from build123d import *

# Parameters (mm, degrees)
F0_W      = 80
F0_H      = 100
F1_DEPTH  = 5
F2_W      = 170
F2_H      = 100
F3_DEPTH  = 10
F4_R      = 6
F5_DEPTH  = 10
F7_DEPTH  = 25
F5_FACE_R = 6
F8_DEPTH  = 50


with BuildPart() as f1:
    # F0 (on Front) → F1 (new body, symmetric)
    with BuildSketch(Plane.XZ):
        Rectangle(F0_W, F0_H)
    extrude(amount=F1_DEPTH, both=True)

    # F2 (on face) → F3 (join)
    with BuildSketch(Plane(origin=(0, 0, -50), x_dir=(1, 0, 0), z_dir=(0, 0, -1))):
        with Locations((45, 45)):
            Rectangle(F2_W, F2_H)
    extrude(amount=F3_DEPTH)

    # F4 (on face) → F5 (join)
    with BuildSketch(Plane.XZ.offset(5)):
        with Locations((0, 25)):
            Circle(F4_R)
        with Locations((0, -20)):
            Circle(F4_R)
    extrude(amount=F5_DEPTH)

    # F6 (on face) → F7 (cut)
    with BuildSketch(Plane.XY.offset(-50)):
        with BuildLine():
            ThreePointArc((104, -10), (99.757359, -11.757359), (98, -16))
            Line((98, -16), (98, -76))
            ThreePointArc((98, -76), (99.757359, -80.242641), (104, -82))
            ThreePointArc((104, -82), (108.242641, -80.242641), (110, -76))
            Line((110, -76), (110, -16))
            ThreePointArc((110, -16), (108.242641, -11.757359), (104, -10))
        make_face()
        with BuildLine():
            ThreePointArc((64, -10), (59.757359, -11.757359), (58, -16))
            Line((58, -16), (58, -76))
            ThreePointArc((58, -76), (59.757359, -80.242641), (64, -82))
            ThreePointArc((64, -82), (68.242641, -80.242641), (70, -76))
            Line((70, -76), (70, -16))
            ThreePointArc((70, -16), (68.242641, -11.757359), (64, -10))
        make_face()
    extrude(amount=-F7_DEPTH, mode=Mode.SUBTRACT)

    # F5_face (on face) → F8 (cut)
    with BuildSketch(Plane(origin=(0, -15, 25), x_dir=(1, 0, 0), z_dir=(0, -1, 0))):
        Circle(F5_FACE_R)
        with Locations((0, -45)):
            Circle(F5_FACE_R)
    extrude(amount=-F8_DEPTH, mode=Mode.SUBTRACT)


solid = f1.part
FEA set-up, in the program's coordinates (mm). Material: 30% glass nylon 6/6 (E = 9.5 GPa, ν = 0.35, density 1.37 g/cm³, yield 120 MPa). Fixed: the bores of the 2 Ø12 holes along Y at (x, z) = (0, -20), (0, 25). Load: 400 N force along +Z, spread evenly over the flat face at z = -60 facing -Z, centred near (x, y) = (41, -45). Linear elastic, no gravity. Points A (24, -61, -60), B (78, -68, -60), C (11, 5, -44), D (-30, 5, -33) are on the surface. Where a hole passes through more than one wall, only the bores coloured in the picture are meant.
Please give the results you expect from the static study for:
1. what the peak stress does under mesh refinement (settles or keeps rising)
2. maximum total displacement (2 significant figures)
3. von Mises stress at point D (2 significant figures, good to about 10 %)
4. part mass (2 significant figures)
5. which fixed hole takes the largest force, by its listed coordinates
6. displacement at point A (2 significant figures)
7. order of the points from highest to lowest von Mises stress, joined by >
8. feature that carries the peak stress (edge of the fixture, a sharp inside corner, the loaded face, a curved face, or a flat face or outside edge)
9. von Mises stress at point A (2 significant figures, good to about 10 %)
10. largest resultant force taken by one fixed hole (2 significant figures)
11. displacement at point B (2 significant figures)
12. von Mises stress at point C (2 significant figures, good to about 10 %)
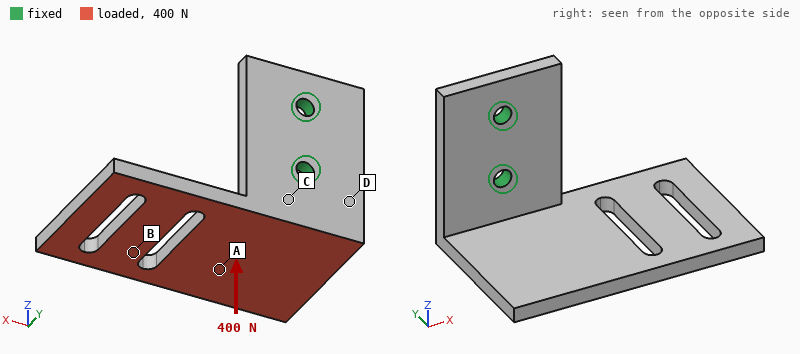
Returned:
keeps rising
2.6 mm
9.4 MPa
320 g
(0, -20)
0.93 mm
C > D > A > B
edge of the fixture
3.7 MPa
420 N
1.5 mm
13 MPa
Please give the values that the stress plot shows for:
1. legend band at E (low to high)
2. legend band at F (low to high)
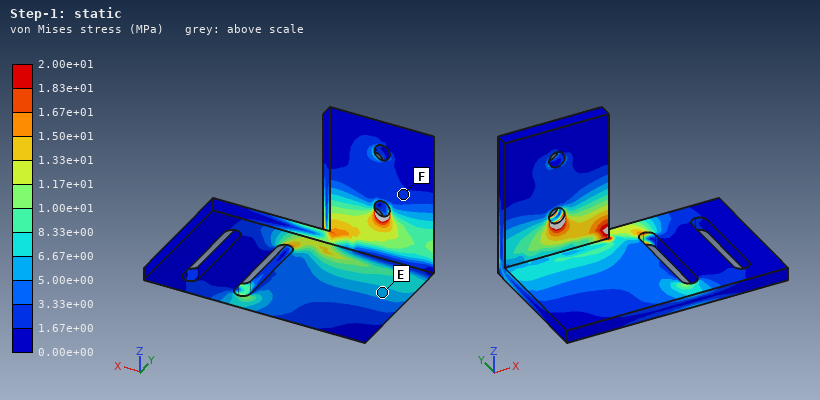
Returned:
5.00e+00 to 6.67e+00 MPa
1.67e+00 to 3.33e+00 MPa
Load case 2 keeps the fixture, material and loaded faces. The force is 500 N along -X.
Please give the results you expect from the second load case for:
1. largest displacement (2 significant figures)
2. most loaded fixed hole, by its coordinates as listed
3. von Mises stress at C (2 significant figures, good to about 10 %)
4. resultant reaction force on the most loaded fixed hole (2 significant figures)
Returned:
1.1 mm
(0, -20)
6.6 MPa
820 N
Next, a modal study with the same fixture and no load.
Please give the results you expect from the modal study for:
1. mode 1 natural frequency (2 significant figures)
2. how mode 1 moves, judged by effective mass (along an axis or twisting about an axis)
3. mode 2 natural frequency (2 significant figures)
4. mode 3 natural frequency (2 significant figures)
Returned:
180 Hz
along Z
250 Hz
330 Hz
